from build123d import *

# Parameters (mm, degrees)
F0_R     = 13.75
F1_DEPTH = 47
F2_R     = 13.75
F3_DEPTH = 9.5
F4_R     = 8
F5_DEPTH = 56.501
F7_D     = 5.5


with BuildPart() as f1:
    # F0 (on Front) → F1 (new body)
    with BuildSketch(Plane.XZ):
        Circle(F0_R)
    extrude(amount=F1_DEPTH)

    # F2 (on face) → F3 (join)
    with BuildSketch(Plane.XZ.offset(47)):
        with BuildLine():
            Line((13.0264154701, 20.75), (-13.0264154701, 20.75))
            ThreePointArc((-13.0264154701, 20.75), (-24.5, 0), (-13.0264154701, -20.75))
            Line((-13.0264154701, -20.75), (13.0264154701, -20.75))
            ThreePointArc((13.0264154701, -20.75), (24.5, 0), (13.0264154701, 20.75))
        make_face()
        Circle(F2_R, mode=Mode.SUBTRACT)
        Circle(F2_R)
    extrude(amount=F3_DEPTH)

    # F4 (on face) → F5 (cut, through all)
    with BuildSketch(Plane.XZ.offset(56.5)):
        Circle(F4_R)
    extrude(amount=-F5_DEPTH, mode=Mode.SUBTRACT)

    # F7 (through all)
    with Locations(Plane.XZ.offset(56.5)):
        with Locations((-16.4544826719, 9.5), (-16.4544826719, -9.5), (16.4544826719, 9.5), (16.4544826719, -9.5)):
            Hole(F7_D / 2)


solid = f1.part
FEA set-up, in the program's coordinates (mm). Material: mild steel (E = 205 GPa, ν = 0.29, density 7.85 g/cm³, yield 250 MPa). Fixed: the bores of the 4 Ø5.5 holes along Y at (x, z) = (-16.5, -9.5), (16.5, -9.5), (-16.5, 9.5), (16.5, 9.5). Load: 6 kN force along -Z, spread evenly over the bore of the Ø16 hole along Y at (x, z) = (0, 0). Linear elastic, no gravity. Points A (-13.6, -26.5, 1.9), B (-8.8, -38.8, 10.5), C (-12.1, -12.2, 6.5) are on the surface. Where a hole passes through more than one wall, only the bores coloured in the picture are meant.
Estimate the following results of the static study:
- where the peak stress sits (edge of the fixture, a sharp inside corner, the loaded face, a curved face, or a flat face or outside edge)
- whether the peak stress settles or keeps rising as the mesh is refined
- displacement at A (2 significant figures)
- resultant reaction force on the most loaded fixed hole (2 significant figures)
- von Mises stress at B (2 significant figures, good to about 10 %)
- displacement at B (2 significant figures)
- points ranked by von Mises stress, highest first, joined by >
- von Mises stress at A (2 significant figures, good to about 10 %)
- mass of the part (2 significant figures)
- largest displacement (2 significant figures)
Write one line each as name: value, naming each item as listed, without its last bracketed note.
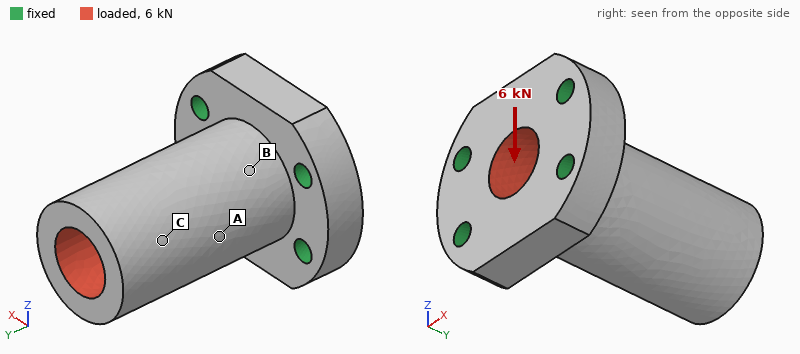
where the peak stress sits: edge of the fixture
whether the peak stress settles or keeps rising as the mesh is refined: keeps rising
displacement at A: 17 µm
resultant reaction force on the most loaded fixed hole: 3.4 kN
von Mises stress at B: 35 MPa
displacement at B: 9.4 µm
points ranked by von Mises stress, highest first, joined by >: B > A > C
von Mises stress at A: 19 MPa
mass of the part: 250 g
largest displacement: 39 µm
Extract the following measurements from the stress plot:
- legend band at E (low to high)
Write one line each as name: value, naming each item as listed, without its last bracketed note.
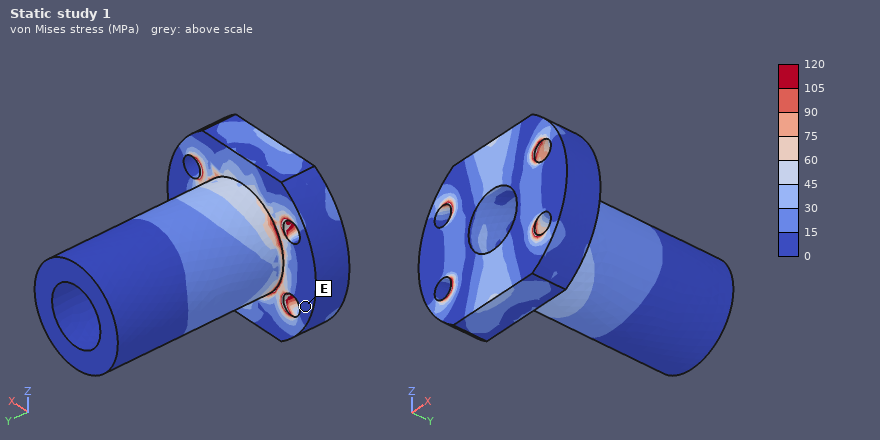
legend band at E: 0 to 15 MPa
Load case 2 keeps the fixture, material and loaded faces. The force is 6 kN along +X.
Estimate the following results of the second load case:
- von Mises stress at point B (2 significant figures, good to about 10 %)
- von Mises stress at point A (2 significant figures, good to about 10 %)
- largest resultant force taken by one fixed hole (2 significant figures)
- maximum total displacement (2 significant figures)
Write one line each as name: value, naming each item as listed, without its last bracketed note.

von Mises stress at point B: 31 MPa
von Mises stress at point A: 20 MPa
largest resultant force taken by one fixed hole: 3.0 kN
maximum total displacement: 29 µm
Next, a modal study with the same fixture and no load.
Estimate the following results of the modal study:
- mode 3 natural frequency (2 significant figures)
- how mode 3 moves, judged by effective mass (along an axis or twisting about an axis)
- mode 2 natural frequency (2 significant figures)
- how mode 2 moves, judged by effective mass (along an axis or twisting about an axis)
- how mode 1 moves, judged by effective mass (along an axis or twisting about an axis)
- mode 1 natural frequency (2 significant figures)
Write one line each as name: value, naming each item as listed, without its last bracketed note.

mode 3 natural frequency: 16 kHz
how mode 3 moves, judged by effective mass: twisting about Y
mode 2 natural frequency: 6600 Hz
how mode 2 moves, judged by effective mass: along X
how mode 1 moves, judged by effective mass: along Z
mode 1 natural frequency: 5600 Hz
